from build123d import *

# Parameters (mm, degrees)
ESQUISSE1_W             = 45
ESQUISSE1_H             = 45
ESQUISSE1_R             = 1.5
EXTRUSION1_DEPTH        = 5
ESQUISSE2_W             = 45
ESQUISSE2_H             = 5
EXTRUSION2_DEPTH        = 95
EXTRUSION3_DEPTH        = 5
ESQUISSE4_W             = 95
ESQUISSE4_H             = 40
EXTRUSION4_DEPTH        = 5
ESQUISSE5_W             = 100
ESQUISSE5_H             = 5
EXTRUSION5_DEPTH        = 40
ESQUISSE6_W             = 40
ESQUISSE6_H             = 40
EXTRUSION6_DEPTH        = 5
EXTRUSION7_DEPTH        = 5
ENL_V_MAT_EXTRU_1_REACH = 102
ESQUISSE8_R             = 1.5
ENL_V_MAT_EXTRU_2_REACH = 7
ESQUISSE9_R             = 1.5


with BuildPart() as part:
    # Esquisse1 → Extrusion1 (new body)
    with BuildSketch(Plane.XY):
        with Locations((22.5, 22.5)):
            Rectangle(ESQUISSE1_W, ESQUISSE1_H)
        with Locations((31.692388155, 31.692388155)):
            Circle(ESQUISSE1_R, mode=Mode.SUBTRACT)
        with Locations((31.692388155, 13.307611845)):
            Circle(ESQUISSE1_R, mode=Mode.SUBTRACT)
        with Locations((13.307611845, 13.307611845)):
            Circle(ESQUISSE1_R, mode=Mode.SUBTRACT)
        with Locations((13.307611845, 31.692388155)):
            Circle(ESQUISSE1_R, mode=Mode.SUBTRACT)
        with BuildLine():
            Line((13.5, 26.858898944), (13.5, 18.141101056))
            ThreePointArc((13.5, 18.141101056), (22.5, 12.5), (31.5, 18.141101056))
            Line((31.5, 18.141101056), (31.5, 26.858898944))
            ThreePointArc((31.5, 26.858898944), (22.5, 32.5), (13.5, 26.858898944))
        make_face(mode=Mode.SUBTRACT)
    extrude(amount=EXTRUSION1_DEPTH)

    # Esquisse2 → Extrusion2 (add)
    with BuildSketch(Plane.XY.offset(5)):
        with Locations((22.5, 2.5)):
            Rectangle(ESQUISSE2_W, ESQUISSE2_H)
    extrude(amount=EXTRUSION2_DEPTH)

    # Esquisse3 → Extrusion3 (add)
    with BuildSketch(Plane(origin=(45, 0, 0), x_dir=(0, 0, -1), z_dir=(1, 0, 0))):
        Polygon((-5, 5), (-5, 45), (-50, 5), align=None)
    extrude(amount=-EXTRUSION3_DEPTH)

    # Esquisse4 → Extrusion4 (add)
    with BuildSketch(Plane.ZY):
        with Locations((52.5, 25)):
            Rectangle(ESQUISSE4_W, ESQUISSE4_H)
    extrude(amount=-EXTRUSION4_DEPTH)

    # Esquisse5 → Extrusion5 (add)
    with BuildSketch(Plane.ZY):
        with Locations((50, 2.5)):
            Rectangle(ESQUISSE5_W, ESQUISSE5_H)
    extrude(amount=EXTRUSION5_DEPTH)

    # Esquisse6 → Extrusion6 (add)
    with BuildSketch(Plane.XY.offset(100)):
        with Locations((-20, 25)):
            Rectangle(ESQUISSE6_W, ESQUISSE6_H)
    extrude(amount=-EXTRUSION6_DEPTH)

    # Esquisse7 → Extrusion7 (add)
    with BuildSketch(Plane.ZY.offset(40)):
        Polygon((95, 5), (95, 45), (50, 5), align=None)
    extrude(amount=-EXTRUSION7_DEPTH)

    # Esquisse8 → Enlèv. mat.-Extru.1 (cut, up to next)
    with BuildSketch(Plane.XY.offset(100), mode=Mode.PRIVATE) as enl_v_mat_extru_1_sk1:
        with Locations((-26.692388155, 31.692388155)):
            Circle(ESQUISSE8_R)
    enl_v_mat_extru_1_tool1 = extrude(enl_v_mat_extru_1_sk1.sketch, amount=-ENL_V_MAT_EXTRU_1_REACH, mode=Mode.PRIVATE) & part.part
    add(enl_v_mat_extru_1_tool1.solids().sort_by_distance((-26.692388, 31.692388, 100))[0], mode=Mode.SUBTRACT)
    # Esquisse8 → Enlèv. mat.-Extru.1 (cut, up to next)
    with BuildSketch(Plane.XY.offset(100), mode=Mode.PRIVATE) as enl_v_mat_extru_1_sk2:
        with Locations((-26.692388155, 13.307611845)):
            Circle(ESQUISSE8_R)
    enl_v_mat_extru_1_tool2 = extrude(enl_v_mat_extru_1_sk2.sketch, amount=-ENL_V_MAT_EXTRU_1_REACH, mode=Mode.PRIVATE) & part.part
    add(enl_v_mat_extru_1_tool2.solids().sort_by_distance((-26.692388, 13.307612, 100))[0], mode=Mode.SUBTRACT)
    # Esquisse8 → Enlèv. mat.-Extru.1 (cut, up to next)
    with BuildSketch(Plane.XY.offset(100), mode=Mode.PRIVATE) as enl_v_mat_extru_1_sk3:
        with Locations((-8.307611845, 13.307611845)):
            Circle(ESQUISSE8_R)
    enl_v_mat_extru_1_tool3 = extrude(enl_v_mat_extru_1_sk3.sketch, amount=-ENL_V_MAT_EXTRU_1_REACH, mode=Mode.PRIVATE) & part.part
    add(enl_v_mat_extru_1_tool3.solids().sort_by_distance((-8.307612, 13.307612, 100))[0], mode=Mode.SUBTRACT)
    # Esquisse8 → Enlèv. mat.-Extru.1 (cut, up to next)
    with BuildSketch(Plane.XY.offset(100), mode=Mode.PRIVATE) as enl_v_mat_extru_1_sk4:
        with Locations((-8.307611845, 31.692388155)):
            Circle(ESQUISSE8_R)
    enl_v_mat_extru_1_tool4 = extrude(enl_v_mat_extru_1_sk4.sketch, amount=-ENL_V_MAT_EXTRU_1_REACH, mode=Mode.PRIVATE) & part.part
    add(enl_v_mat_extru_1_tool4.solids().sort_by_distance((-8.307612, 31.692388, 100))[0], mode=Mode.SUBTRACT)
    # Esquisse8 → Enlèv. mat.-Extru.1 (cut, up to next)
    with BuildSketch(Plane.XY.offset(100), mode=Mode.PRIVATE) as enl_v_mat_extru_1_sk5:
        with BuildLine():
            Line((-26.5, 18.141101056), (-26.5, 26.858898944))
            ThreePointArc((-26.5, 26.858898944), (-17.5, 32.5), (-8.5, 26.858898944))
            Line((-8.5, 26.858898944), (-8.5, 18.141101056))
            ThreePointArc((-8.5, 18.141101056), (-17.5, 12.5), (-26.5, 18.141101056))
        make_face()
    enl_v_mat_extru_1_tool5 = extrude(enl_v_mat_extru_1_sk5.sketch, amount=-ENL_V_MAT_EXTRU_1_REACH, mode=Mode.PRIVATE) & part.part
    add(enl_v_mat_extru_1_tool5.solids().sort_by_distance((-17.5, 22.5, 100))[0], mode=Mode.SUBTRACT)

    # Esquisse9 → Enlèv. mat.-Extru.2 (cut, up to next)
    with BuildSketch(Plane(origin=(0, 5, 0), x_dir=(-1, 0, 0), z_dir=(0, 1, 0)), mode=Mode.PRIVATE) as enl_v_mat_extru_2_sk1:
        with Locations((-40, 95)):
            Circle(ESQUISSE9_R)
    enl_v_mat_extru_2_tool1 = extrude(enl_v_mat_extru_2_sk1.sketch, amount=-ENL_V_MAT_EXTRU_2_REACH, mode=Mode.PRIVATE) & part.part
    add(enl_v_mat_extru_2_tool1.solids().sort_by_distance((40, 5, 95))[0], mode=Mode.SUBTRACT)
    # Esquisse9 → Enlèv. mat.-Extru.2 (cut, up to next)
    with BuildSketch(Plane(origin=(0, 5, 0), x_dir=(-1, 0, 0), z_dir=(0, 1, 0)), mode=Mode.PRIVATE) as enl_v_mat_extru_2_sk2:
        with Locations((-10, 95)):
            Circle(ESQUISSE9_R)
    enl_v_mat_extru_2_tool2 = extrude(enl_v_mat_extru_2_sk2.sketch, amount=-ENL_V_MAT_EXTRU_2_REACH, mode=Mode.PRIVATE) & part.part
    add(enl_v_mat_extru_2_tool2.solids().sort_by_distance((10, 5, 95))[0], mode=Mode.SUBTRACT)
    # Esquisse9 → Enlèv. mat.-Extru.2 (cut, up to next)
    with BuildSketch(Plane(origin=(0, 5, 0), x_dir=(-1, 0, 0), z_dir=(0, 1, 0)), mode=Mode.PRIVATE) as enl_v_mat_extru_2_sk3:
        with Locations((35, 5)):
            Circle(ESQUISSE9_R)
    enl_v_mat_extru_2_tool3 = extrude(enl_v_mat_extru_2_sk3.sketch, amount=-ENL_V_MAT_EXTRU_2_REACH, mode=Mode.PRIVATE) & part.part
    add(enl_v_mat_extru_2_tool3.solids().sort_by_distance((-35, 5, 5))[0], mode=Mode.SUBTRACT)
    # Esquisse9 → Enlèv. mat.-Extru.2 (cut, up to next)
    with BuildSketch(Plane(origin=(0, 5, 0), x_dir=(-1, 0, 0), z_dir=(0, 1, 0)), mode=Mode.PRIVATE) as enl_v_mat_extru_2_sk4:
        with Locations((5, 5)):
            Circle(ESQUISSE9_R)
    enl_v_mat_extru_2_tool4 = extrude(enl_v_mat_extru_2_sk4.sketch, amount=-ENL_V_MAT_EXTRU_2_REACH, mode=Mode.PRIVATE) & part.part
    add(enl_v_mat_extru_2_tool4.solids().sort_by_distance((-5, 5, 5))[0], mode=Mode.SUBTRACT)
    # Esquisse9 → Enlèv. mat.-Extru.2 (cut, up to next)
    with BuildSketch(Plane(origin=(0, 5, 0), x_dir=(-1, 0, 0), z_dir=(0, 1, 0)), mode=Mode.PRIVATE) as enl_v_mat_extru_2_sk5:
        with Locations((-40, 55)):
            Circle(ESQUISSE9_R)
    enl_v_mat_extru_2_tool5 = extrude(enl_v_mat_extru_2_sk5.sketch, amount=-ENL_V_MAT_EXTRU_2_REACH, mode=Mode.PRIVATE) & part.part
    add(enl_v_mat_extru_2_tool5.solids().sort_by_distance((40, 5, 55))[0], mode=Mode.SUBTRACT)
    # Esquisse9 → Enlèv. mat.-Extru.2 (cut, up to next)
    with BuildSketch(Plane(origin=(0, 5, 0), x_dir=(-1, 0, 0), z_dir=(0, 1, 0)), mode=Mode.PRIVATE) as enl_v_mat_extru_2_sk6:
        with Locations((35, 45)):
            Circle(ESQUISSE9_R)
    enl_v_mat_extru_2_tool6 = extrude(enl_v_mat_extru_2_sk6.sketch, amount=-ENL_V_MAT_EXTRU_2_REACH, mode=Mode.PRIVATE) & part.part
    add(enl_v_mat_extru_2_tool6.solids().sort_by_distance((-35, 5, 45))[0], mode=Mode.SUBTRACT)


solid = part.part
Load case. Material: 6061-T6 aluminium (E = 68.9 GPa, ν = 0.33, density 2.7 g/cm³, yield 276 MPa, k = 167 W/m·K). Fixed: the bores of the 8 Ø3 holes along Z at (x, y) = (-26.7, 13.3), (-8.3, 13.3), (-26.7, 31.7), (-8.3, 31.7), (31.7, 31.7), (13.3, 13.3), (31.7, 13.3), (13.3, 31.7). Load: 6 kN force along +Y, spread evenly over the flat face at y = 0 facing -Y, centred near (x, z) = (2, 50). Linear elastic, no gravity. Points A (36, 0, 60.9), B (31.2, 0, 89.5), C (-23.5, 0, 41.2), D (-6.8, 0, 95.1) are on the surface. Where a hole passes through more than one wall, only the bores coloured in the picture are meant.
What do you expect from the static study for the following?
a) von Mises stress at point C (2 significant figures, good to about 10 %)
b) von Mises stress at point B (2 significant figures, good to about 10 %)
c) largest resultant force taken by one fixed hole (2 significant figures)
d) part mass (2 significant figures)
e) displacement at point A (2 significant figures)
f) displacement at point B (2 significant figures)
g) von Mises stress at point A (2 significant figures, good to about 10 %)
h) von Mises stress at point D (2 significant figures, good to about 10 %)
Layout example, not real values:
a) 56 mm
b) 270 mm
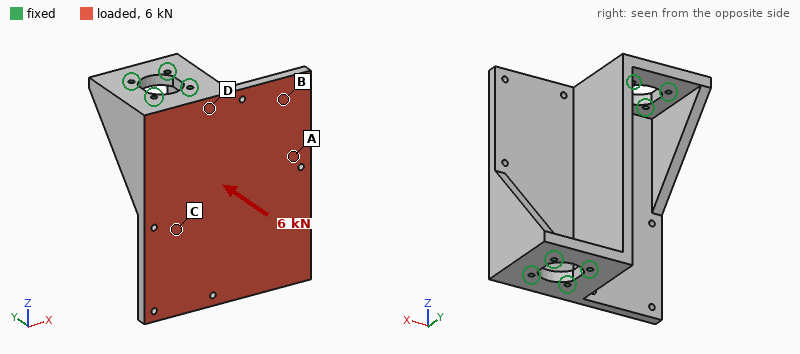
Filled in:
a) 38 MPa
b) 25 MPa
c) 1.1 kN
d) 230 g
e) 0.10 mm
f) 0.16 mm
g) 44 MPa
h) 15 MPa
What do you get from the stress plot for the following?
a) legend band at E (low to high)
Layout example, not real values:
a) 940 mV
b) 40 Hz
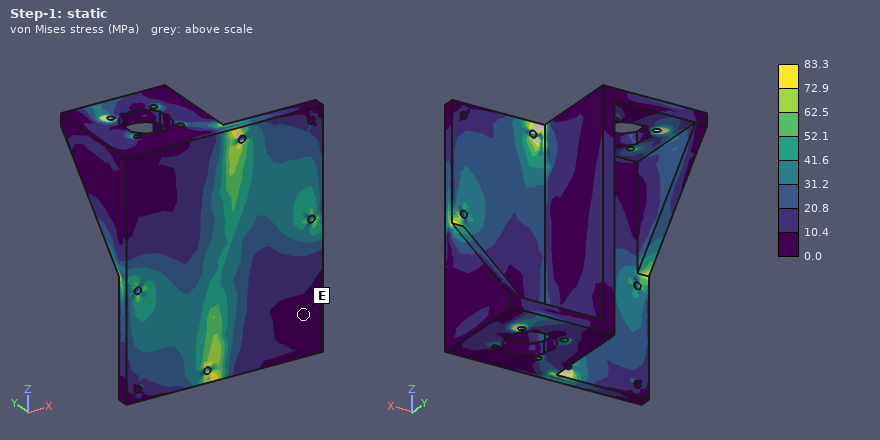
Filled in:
a) 0.0 to 10.4 MPa
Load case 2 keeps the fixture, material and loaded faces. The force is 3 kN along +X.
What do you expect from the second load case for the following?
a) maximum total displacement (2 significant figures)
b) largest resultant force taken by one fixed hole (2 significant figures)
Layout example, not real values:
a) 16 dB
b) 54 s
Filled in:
a) 38 µm
b) 1.0 kN
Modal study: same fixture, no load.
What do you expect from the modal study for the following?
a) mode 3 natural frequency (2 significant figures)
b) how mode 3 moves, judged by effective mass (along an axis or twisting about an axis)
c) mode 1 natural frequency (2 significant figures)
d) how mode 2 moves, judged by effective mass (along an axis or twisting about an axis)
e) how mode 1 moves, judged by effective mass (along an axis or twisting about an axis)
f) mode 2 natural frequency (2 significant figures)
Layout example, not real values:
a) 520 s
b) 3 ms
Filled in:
a) 3800 Hz
b) along X
c) 2900 Hz
d) along Y
e) twisting about Z
f) 3100 Hz
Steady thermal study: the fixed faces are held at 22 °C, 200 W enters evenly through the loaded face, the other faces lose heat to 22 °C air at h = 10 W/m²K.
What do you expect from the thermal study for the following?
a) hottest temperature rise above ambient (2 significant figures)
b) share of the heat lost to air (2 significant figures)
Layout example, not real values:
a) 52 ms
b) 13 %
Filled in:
a) 58 K
b) 3.9 %
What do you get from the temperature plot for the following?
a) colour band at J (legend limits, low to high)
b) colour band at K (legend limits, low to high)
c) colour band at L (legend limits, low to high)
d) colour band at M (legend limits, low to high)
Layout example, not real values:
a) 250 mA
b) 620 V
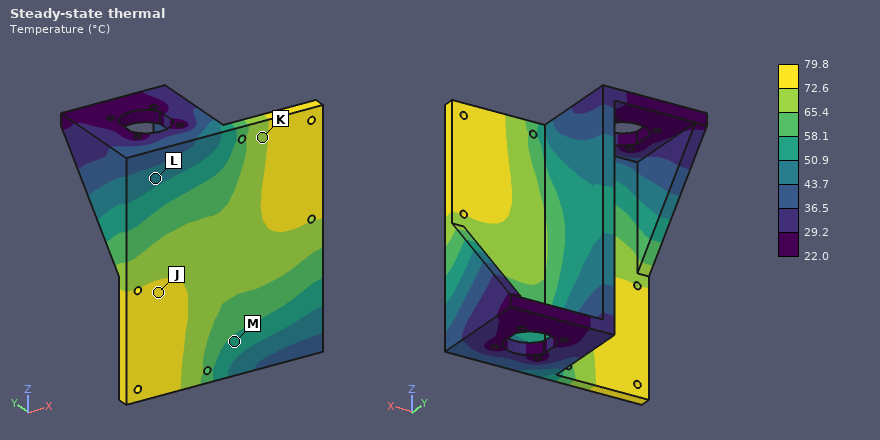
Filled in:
a) 72.6 to 79.8 °C
b) 65.4 to 72.6 °C
c) 43.7 to 50.9 °C
d) 50.9 to 58.1 °C
